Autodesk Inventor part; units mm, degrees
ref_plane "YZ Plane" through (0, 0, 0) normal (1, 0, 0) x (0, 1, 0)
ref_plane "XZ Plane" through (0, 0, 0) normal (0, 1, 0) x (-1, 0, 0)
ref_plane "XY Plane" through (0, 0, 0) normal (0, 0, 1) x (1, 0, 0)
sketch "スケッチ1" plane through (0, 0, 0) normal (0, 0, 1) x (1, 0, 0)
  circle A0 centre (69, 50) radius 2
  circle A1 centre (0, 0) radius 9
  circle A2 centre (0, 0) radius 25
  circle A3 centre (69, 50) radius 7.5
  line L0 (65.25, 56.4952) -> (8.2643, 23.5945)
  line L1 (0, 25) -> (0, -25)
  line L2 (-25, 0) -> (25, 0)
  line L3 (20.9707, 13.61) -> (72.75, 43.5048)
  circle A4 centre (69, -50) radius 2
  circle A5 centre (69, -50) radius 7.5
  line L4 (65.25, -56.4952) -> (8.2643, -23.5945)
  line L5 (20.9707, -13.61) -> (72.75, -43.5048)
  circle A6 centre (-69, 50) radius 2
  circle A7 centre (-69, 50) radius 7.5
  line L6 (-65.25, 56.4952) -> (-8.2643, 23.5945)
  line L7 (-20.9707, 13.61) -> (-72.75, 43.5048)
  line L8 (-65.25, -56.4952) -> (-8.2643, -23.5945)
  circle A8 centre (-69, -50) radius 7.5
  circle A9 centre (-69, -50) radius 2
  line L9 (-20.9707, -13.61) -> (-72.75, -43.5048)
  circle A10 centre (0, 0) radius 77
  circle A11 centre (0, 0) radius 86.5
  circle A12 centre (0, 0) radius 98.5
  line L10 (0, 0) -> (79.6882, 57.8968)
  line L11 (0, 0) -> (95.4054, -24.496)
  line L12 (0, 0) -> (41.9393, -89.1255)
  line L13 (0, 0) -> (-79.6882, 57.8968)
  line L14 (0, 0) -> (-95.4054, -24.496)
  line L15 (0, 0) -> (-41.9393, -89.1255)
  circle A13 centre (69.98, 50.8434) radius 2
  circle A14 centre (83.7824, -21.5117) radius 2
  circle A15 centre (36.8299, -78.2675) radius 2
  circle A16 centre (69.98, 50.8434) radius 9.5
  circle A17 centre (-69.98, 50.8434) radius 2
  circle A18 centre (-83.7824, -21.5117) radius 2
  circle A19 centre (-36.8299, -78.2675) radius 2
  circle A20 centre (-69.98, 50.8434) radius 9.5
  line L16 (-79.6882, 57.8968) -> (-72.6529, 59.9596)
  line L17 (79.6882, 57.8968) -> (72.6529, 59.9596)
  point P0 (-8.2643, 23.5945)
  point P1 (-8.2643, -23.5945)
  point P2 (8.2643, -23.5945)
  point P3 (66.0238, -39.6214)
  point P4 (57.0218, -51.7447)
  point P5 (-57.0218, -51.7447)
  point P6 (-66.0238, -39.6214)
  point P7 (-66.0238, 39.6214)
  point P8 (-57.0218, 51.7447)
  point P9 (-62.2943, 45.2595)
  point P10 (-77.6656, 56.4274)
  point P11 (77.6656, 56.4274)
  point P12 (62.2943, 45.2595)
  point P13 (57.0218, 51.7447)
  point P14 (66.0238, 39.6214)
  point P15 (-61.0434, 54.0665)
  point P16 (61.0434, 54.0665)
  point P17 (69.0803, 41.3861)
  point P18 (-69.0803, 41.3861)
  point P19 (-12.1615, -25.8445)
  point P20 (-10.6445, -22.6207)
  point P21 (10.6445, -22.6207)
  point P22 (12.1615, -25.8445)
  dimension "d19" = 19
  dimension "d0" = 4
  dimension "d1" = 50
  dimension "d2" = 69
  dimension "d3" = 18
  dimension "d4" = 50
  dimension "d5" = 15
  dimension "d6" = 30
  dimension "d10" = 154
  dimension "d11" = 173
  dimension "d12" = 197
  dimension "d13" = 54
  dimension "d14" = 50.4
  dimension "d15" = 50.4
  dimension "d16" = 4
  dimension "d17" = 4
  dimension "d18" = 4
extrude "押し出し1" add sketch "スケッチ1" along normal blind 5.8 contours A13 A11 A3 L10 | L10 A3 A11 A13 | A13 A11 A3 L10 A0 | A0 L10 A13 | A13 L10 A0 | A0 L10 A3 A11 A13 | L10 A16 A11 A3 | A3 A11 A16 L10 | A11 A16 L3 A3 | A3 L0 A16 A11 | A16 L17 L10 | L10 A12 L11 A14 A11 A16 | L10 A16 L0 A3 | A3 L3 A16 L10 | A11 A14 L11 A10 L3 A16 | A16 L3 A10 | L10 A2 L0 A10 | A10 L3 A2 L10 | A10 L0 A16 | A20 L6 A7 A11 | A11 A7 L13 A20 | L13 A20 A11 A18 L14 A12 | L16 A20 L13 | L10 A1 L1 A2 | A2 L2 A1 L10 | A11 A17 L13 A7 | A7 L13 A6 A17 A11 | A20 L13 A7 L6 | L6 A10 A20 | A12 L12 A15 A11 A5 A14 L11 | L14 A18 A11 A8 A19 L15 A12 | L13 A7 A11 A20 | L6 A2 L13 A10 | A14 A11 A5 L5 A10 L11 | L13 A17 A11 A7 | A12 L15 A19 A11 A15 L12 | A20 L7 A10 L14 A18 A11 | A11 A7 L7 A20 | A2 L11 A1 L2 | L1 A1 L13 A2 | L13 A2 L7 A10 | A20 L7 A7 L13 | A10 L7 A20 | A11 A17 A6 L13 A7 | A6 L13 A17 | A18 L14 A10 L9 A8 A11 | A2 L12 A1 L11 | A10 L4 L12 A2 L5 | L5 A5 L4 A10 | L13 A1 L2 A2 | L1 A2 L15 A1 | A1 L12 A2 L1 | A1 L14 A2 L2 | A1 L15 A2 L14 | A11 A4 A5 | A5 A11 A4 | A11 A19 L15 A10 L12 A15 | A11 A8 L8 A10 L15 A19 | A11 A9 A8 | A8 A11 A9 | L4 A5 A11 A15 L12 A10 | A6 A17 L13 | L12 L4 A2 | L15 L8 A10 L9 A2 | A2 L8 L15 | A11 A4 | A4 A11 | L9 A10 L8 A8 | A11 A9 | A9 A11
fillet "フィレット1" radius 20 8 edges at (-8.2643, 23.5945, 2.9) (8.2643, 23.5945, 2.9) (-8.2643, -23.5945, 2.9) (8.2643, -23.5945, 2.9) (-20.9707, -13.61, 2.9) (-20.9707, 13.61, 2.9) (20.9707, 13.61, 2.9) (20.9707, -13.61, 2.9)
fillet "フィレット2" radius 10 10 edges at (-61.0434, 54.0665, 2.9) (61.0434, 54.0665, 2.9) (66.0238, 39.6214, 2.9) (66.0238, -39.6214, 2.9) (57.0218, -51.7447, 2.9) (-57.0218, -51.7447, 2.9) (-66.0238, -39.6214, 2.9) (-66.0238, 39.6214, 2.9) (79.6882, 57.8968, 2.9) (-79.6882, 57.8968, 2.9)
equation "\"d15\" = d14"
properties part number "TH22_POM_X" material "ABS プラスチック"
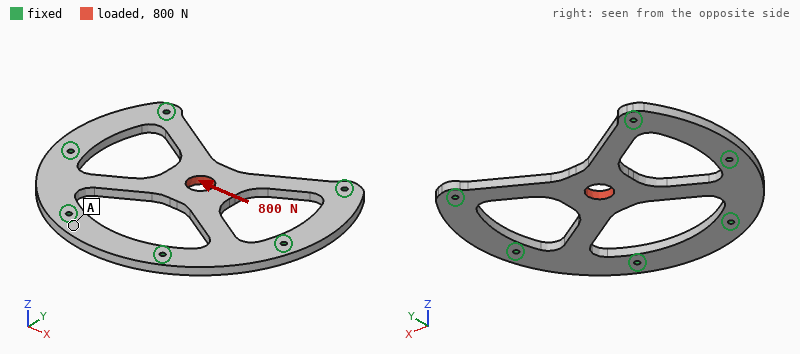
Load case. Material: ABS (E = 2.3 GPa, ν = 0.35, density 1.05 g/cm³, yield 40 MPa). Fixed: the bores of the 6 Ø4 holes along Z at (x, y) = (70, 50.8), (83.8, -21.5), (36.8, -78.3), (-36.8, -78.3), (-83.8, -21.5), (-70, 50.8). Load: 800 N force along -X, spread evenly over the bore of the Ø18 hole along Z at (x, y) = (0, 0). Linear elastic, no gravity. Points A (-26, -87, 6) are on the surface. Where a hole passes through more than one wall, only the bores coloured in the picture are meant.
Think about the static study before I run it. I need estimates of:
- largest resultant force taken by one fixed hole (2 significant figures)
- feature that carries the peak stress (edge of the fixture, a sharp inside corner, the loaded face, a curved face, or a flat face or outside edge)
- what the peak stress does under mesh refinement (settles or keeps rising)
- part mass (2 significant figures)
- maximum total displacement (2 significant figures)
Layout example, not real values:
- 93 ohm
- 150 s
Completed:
- 260 N
- edge of the fixture
- keeps rising
- 84 g
- 0.14 mm
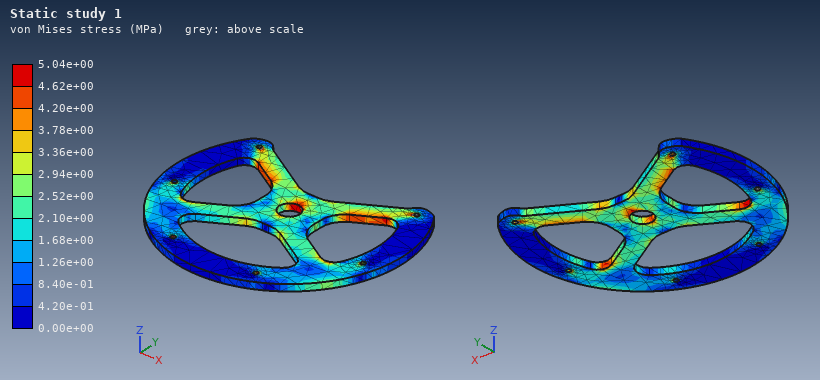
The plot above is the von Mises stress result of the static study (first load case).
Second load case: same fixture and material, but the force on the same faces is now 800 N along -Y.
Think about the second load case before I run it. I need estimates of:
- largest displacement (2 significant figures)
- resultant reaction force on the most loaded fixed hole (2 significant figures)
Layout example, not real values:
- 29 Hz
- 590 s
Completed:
- 0.28 mm
- 400 N
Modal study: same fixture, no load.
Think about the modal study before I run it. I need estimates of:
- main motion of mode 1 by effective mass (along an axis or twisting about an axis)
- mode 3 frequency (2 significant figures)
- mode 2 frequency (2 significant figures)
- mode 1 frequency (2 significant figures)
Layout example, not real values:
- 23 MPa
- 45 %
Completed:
- along Z
- 830 Hz
- 740 Hz
- 320 Hz
